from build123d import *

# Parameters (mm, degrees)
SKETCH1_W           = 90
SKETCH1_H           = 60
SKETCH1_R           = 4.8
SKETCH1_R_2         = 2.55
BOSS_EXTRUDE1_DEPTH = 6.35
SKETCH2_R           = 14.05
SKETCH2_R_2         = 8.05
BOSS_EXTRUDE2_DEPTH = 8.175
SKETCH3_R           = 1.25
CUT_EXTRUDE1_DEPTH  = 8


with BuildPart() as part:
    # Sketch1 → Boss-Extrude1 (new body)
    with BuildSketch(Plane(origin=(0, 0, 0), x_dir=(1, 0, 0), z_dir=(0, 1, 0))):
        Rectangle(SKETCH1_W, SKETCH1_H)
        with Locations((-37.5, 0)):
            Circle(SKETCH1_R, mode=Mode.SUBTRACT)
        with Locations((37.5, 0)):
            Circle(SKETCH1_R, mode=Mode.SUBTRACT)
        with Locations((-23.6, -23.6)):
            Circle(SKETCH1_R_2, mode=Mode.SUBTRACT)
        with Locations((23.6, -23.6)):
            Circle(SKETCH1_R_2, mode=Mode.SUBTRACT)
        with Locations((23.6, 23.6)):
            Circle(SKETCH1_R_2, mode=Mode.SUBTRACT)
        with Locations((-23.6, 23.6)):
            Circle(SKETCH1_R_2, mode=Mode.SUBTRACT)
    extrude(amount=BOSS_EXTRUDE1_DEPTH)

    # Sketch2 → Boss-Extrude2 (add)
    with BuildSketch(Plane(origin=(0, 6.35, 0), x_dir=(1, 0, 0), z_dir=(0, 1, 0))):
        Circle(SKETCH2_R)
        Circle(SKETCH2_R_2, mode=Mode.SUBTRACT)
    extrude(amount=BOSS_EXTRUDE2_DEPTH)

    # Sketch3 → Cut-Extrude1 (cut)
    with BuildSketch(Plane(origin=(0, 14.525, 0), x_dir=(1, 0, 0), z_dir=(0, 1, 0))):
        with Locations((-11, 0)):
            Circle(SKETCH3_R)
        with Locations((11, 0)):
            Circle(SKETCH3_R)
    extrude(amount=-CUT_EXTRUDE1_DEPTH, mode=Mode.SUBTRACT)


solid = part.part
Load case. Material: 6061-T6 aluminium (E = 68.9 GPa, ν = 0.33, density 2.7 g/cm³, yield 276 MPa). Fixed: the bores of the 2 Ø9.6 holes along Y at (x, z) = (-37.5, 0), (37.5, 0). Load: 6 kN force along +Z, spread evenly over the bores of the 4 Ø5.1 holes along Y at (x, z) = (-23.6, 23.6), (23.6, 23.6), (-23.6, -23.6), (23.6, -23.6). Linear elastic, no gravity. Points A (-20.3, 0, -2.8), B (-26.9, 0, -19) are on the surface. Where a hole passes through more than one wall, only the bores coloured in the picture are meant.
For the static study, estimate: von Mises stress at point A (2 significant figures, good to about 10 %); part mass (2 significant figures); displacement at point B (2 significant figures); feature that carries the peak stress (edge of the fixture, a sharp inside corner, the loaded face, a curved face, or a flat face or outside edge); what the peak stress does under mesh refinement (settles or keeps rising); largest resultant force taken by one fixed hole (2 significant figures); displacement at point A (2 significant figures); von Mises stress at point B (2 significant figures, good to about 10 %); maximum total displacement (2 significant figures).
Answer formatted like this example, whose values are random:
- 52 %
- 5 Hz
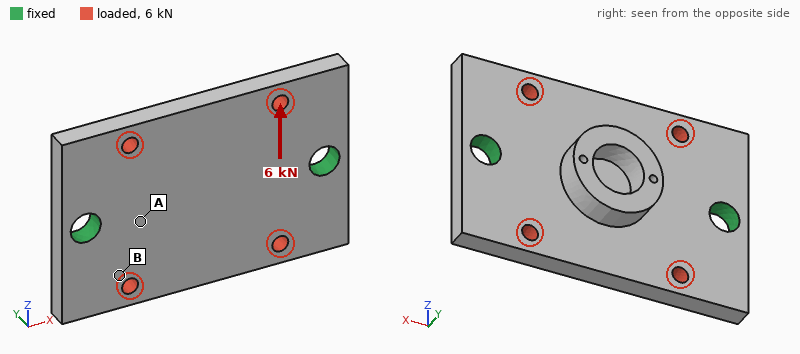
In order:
- 6.6 MPa
- 98 g
- 6.0 µm
- edge of the fixture
- keeps rising
- 3.0 kN
- 6.2 µm
- 15 MPa
- 9.4 µm
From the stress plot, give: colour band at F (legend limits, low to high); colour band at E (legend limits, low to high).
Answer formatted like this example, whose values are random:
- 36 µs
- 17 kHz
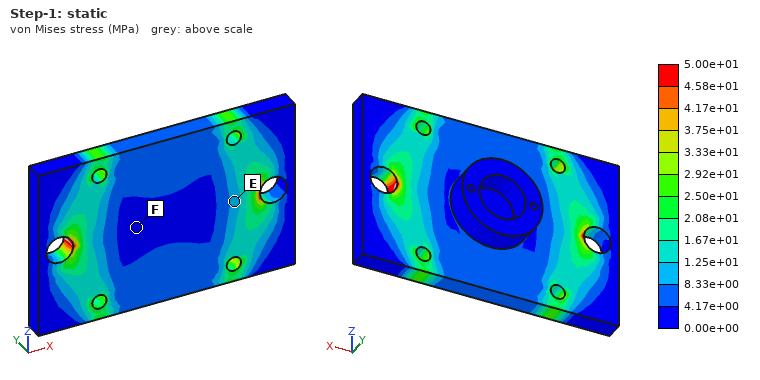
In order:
- 0.00e+00 to 4.17e+00 MPa
- 8.33e+00 to 1.25e+01 MPa
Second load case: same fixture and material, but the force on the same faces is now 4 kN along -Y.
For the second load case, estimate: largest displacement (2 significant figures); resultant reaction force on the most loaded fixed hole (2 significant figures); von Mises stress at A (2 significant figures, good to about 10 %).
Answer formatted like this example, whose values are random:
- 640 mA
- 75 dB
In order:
- 92 µm
- 2.0 kN
- 41 MPa
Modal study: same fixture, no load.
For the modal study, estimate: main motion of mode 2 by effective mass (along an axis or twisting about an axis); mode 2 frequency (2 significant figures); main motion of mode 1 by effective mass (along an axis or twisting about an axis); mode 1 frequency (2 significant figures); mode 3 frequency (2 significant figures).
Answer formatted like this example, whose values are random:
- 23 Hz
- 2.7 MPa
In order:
- along Y
- 4800 Hz
- twisting about X
- 3900 Hz
- 8000 Hz
